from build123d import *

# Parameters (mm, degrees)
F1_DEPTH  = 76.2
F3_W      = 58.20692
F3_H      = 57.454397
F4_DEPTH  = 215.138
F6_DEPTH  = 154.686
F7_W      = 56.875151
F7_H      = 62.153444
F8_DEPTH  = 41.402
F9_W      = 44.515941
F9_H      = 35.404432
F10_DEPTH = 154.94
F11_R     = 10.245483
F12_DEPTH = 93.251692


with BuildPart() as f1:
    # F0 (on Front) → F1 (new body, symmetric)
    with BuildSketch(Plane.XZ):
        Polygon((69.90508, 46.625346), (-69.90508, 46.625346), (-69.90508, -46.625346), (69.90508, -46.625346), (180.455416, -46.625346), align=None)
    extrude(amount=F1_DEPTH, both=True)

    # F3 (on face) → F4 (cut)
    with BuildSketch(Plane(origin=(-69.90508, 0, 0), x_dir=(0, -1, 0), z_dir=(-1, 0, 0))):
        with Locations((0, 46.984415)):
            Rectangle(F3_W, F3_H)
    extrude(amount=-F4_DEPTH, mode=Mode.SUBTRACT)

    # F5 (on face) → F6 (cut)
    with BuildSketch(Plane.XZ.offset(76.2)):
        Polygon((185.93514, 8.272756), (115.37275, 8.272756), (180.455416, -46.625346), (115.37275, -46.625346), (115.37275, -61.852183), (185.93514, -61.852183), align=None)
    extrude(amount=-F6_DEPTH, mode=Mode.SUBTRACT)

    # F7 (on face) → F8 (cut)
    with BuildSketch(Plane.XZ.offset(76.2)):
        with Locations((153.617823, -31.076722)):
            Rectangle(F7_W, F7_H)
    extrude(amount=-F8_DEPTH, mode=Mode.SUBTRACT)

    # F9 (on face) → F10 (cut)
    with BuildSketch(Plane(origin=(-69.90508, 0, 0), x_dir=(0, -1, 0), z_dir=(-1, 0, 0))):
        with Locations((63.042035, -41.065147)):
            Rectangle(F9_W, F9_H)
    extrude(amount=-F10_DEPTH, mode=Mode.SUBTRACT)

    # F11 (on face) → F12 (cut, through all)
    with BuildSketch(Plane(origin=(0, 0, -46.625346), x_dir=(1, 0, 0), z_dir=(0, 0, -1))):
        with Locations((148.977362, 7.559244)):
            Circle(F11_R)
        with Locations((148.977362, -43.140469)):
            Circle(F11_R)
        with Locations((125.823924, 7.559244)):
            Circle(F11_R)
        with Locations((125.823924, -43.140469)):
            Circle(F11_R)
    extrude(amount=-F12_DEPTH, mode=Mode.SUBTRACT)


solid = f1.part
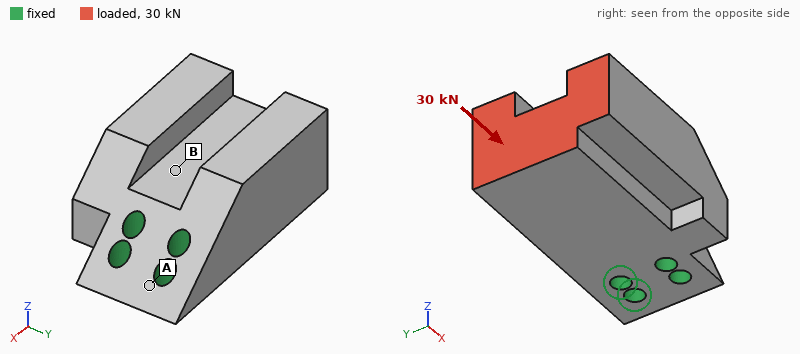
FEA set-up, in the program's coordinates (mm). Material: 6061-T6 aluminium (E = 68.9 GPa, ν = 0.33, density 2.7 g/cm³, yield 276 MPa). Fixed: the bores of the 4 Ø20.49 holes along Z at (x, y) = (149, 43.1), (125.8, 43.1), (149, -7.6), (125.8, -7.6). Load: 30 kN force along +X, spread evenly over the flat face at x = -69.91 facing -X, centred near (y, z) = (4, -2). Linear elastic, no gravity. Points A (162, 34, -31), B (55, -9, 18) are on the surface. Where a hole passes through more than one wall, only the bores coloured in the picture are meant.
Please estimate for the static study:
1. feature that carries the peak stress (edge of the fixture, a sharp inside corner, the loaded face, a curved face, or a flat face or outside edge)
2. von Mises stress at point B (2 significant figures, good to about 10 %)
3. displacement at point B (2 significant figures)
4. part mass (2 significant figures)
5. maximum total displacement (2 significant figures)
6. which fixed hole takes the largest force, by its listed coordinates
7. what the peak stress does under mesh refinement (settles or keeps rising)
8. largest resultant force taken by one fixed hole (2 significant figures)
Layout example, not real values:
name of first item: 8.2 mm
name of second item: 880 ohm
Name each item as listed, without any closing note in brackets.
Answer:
feature that carries the peak stress: edge of the fixture
von Mises stress at point B: 5.3 MPa
displacement at point B: 16 µm
part mass: 6.2 kg
maximum total displacement: 45 µm
which fixed hole takes the largest force, by its listed coordinates: (125.8, -7.6)
what the peak stress does under mesh refinement: keeps rising
largest resultant force taken by one fixed hole: 19 kN
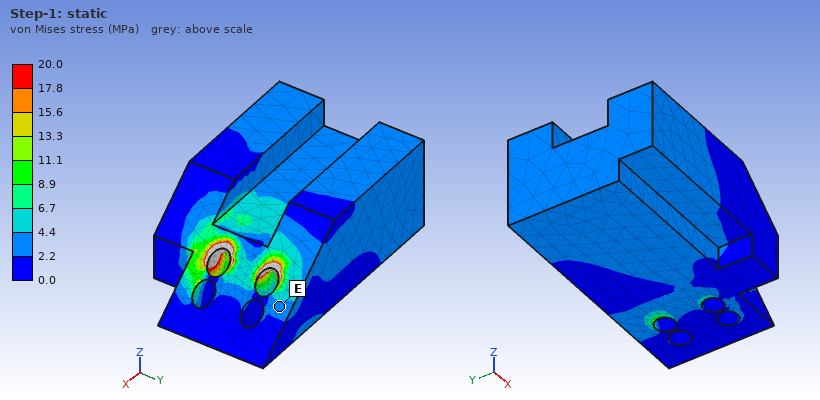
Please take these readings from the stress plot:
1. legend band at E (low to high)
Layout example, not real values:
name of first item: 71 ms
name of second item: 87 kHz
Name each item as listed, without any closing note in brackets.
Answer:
legend band at E: 2.2 to 4.4 MPa
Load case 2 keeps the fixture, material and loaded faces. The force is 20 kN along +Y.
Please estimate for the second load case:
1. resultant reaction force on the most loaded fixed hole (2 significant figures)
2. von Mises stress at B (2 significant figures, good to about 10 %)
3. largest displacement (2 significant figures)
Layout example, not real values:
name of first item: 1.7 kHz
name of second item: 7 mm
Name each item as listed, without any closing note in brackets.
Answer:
resultant reaction force on the most loaded fixed hole: 52 kN
von Mises stress at B: 7.7 MPa
largest displacement: 0.14 mm
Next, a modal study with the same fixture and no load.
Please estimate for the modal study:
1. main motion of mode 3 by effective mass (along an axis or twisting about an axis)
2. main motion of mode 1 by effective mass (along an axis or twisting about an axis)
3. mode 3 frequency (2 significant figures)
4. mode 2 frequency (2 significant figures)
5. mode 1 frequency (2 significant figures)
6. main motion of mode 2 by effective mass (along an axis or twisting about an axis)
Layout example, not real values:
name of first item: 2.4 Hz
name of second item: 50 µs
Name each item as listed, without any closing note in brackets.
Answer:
main motion of mode 3 by effective mass: twisting about X
main motion of mode 1 by effective mass: along Z
mode 3 frequency: 2100 Hz
mode 2 frequency: 1400 Hz
mode 1 frequency: 960 Hz
main motion of mode 2 by effective mass: along Y
